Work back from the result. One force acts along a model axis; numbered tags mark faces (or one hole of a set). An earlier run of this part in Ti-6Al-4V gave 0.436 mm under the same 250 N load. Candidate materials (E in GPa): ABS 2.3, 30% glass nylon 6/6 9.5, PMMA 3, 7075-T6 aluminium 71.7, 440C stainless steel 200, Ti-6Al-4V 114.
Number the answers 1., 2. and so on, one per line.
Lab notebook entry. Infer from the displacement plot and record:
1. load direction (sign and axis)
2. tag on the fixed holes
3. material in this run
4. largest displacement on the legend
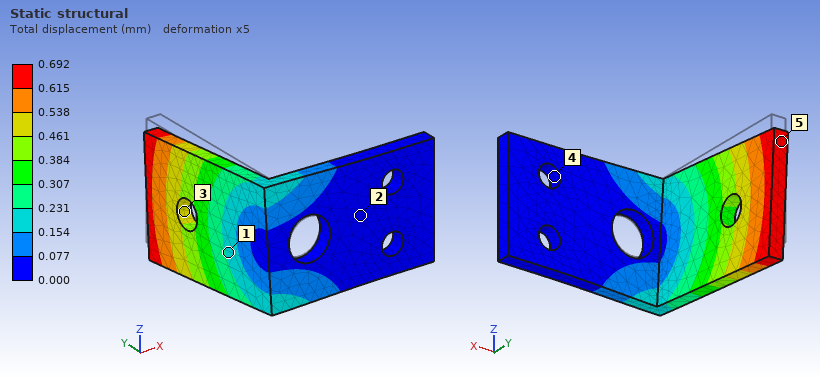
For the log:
1. -Z
2. 4
3. 7075-T6 aluminium
4. 0.692 mm
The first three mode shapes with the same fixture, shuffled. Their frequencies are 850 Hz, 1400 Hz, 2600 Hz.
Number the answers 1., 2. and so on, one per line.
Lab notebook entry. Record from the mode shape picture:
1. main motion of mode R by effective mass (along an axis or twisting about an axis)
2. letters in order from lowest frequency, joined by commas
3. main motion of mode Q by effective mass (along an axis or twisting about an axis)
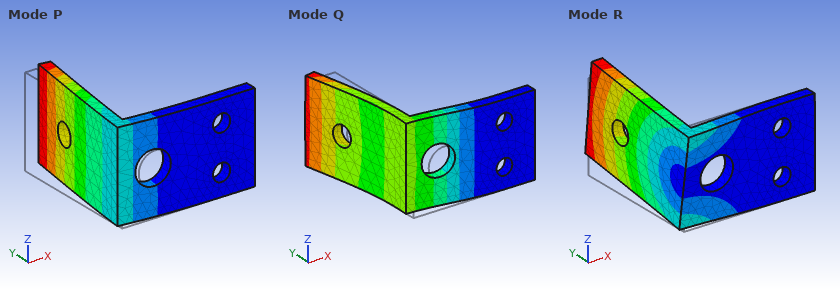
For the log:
1. along Z
2. P, R, Q
3. along Y
